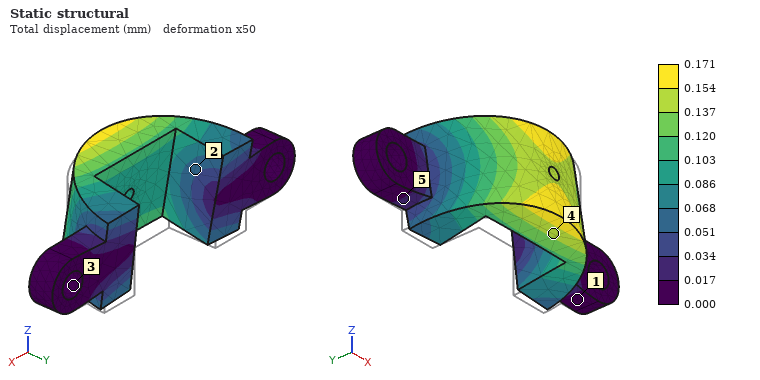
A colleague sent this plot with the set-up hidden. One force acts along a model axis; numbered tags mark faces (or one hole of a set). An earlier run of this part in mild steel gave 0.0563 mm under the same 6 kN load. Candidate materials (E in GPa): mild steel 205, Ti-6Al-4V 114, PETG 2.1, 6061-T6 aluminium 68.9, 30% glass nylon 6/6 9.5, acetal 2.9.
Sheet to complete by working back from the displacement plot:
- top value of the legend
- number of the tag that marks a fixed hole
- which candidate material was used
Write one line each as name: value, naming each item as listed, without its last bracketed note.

top value of the legend: 0.171 mm
number of the tag that marks a fixed hole: 3
which candidate material was used: 6061-T6 aluminium
